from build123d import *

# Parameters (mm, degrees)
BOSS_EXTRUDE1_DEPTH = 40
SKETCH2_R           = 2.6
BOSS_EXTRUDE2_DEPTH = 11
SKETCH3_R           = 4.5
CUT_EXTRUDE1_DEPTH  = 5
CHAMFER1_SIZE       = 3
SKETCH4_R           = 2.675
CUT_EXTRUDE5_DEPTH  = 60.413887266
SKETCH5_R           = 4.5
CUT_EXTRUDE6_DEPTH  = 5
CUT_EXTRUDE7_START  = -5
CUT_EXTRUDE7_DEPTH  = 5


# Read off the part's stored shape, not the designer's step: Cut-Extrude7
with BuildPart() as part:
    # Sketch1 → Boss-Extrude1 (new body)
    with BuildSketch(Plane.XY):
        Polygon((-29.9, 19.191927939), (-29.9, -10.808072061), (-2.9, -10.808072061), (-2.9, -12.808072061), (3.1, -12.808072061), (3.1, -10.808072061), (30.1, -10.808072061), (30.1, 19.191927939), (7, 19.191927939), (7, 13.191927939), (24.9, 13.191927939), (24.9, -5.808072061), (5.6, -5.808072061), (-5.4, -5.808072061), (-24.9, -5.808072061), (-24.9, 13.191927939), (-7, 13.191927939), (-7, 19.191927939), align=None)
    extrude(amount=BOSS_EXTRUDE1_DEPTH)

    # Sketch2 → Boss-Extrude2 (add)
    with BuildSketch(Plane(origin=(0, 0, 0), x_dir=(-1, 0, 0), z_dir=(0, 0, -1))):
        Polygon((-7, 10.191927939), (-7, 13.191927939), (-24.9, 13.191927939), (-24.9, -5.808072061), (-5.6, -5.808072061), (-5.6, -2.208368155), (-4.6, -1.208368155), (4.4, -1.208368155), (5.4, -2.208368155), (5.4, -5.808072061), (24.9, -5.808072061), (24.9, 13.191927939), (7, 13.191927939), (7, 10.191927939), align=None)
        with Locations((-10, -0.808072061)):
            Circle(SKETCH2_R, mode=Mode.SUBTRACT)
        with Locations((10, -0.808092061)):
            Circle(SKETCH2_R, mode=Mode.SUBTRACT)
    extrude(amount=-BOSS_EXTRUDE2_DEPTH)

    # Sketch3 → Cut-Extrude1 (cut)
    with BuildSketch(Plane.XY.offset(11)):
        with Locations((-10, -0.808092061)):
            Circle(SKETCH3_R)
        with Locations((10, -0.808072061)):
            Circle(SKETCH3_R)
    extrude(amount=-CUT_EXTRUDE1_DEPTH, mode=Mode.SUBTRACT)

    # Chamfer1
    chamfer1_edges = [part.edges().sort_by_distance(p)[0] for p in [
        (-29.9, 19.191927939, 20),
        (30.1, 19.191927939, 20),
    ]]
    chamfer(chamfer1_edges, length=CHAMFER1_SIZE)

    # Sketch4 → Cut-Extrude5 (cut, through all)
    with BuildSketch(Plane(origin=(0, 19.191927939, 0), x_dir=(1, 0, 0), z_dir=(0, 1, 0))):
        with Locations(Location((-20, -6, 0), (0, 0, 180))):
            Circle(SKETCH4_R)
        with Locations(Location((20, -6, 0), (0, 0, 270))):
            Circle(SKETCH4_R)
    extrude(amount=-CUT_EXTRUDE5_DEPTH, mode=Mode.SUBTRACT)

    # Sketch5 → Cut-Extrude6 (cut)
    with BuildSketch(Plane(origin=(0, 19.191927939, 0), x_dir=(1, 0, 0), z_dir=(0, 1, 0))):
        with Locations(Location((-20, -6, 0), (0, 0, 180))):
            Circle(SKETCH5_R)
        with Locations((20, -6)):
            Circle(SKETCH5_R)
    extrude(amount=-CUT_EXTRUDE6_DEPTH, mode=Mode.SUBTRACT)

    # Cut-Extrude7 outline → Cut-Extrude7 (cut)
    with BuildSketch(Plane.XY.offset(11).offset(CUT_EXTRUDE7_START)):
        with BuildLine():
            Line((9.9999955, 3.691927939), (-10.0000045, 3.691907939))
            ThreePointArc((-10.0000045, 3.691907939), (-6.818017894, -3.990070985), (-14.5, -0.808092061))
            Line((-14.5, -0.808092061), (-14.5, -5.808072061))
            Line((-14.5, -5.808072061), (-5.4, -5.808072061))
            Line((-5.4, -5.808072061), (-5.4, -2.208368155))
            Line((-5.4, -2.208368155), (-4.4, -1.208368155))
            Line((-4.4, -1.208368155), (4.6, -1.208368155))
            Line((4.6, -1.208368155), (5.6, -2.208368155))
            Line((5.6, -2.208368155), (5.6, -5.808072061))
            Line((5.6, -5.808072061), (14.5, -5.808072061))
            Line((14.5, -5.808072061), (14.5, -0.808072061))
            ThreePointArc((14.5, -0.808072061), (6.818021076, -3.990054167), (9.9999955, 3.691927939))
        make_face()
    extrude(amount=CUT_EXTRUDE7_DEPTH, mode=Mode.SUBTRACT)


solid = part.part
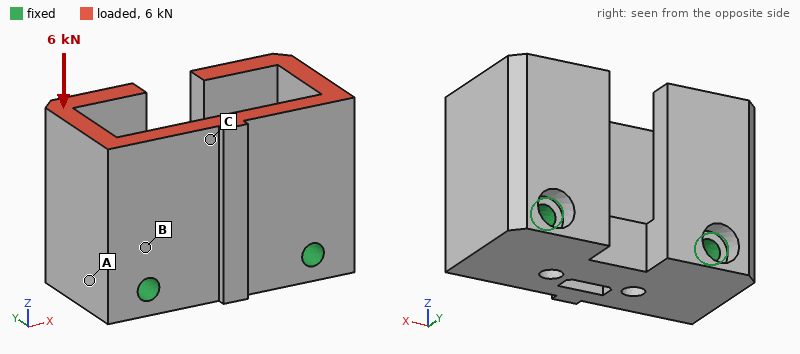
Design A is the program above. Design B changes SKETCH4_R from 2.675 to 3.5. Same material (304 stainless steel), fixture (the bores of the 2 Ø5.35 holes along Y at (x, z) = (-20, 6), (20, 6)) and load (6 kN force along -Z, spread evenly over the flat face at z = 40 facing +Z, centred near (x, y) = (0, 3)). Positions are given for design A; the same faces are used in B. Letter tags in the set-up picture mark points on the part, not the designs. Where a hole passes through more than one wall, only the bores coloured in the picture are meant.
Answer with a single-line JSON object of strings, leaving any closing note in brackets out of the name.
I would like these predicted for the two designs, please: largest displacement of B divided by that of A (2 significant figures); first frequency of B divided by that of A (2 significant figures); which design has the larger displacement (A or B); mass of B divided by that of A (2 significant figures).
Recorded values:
{"largest displacement of B divided by that of A": "0.90", "first frequency of B divided by that of A": "1.1", "which design has the larger displacement": "A", "mass of B divided by that of A": "0.98"}
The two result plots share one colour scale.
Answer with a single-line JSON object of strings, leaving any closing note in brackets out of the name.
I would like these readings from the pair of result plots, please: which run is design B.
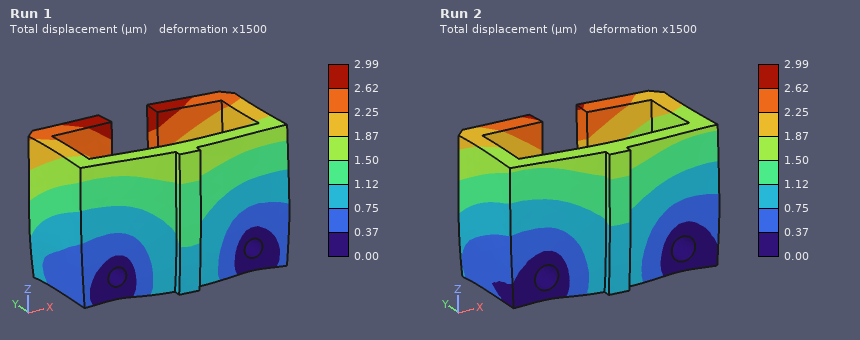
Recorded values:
{"which run is design B": "Run 2"}
